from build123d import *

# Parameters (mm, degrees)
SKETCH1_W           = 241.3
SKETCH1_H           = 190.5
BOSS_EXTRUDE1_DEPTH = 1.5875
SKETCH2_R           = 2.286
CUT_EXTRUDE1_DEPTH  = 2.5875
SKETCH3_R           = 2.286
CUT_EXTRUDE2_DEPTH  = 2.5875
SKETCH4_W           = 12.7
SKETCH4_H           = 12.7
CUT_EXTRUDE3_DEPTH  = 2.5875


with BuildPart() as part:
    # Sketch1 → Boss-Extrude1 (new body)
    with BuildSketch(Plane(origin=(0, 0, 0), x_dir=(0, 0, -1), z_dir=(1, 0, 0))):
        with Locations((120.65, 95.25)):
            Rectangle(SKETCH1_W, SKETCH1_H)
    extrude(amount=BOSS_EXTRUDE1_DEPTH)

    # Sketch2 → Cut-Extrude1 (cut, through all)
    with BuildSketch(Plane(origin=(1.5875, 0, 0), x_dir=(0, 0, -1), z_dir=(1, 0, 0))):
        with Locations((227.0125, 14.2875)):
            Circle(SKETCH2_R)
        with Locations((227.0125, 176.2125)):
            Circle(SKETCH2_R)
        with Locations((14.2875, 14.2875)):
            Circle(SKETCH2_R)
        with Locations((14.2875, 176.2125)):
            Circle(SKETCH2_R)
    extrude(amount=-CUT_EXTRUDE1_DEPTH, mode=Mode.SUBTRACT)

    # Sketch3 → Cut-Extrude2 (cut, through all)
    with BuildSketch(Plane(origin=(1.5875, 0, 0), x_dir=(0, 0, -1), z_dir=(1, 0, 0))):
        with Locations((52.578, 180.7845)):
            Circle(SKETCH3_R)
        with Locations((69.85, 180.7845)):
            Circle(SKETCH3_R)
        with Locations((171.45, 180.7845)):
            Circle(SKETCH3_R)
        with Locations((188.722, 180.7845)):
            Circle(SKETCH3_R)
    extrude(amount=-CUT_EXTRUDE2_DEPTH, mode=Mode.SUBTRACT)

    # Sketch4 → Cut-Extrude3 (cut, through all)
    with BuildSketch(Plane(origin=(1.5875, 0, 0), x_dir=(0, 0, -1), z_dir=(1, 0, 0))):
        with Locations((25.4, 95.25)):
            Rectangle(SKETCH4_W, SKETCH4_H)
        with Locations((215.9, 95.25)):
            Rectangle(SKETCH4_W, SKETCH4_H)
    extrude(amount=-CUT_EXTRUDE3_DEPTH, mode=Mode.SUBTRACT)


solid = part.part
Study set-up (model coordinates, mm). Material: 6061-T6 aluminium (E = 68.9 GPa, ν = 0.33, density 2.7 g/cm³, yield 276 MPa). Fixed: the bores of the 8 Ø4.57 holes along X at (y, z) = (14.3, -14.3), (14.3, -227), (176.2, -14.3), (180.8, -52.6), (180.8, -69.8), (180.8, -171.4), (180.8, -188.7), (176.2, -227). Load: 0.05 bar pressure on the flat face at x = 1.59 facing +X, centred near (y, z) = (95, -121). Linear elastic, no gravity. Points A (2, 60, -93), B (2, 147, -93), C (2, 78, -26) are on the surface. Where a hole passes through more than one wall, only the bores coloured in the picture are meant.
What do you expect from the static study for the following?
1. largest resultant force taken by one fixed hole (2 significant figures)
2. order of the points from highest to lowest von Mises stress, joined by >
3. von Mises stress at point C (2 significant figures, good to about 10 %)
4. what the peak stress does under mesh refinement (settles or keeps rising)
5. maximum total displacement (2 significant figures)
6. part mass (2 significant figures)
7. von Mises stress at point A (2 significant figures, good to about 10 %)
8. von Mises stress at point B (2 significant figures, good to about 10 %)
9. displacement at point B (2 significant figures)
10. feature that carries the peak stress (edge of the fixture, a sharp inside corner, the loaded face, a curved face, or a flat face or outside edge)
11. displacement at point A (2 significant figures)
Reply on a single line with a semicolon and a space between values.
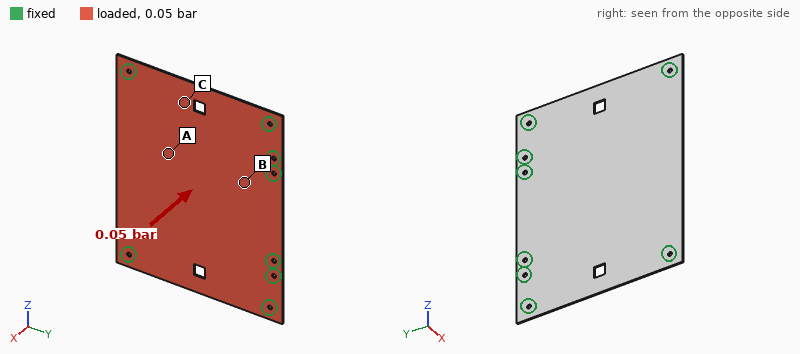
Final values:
53 N; A > C > B; 15 MPa; keeps rising; 1.5 mm; 200 g; 18 MPa; 5.7 MPa; 0.45 mm; edge of the fixture; 1.3 mm
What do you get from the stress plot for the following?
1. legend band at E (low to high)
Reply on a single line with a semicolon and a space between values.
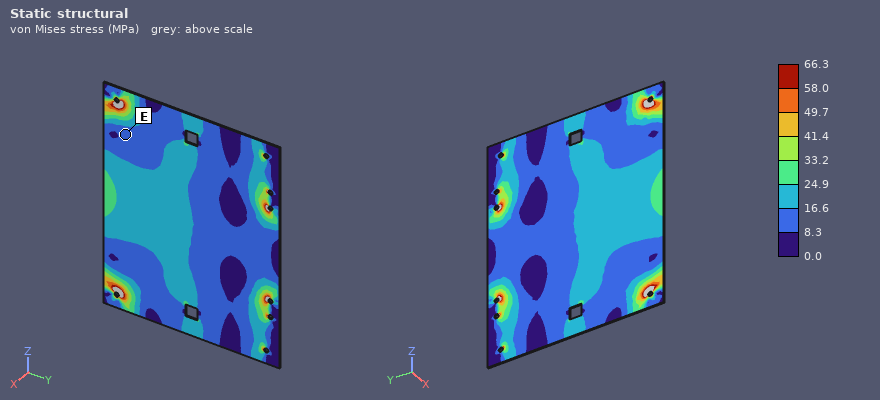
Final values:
8.3 to 16.6 MPa
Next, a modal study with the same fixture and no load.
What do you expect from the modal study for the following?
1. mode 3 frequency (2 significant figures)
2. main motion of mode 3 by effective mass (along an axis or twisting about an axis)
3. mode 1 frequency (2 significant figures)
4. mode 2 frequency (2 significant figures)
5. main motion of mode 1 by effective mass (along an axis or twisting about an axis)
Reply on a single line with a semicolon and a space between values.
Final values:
320 Hz; twisting about Y; 170 Hz; 300 Hz; along X
